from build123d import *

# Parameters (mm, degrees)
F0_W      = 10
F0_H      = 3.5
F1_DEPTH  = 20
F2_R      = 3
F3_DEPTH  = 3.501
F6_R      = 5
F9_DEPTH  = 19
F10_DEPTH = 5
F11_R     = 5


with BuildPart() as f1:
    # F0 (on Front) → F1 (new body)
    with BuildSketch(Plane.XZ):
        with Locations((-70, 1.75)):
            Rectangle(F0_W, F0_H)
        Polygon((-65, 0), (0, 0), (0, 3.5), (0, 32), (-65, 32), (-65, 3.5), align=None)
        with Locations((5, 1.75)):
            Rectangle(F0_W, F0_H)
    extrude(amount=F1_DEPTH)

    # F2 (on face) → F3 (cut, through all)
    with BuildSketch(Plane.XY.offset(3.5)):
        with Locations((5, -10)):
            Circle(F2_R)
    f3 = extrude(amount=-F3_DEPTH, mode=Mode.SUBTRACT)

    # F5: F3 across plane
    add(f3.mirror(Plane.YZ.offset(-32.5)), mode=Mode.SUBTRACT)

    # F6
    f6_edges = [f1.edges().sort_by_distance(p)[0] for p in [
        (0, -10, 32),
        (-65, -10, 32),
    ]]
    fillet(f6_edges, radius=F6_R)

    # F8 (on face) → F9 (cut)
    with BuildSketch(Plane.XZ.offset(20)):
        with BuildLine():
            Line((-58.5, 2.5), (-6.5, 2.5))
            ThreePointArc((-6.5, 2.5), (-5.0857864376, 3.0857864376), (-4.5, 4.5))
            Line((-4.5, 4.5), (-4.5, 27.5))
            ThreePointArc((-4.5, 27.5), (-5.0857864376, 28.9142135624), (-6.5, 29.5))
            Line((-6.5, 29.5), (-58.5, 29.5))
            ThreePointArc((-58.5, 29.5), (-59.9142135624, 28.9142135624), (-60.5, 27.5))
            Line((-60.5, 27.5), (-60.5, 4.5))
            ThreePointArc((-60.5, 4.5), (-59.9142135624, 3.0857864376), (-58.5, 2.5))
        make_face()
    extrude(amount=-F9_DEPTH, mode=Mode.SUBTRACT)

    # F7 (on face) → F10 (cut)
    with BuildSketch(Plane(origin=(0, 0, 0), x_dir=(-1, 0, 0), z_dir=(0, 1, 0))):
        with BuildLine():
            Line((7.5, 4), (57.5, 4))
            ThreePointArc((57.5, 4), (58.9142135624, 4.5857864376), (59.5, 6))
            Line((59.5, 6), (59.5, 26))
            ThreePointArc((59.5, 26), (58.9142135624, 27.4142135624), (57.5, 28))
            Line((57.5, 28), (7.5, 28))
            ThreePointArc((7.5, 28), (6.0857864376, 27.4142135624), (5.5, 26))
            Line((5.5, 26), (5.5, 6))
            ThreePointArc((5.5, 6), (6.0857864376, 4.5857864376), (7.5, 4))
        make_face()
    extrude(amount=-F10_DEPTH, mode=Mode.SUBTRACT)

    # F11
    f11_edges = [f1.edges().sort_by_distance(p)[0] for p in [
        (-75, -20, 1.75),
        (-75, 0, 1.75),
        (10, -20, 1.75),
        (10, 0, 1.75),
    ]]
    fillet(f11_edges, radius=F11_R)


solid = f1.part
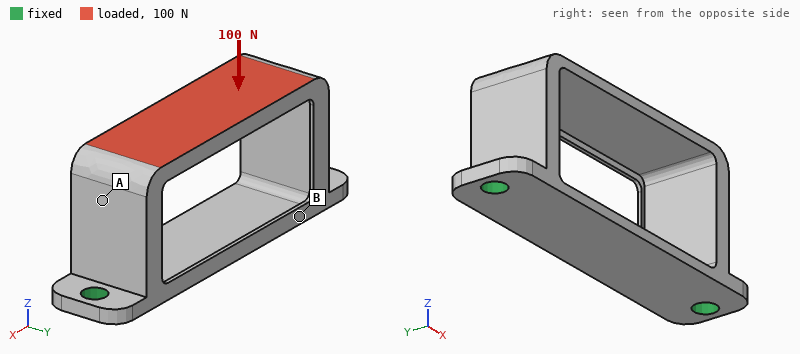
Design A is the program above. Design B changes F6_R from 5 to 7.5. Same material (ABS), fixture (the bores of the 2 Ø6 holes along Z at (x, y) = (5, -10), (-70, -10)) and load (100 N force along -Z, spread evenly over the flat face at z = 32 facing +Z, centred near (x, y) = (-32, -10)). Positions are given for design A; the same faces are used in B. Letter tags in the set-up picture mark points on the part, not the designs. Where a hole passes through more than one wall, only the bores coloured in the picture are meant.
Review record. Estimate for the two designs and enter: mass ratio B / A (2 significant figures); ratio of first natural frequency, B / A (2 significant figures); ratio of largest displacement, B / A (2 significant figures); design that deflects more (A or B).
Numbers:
0.98
1.0
1.2
B
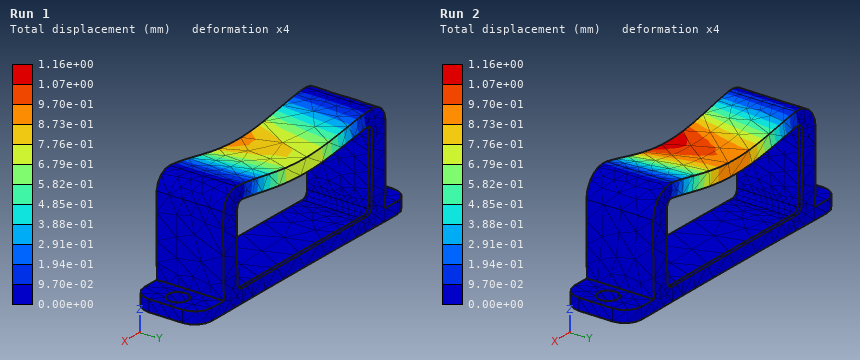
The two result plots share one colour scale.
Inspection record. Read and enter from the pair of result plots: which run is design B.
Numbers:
Run 2
